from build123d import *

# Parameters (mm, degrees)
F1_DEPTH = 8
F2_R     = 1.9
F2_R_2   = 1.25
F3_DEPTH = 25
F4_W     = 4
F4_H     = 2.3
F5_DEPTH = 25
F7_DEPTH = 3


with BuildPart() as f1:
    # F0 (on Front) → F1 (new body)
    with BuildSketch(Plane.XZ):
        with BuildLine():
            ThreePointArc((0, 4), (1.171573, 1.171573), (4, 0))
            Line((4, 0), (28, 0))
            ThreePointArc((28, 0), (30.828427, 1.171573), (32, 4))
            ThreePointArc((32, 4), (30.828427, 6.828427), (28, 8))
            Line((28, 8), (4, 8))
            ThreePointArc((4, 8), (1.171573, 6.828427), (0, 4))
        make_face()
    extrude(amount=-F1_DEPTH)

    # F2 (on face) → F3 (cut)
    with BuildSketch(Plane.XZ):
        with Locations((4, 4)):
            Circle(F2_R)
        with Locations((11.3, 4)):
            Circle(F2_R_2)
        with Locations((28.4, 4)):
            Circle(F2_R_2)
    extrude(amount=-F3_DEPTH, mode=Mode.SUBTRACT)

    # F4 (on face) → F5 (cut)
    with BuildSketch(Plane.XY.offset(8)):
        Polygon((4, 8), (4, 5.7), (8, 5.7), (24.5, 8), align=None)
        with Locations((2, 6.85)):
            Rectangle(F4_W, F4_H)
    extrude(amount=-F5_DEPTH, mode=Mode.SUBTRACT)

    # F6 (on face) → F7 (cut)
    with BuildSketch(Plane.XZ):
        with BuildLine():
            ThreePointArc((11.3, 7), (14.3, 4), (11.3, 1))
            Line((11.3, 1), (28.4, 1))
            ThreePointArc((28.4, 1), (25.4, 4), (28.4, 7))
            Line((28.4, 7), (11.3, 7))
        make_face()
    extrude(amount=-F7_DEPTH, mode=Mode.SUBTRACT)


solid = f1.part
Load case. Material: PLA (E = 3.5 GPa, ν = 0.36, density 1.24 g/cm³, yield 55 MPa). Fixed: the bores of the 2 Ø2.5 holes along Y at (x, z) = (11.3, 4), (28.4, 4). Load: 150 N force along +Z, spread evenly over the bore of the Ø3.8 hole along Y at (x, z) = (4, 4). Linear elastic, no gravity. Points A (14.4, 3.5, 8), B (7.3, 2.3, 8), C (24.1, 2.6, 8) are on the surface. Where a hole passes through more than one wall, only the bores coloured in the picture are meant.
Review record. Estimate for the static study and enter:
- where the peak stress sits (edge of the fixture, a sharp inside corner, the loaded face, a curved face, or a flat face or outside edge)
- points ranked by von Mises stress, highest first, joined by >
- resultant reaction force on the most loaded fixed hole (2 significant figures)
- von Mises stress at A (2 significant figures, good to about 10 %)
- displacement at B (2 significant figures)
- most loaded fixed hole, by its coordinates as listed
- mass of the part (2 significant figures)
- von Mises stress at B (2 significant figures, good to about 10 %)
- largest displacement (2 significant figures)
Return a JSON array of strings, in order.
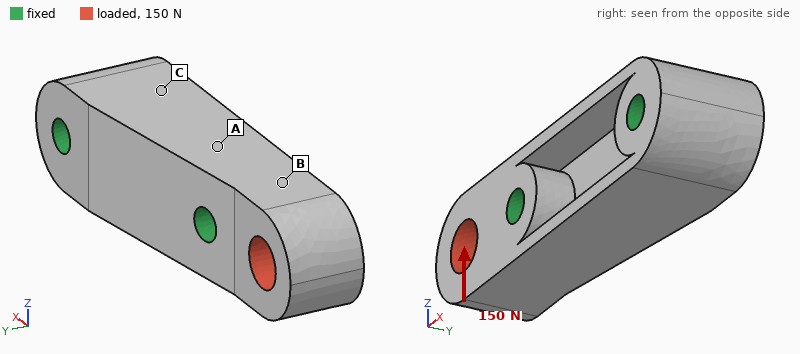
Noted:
["edge of the fixture", "B > A > C", "180 N", "6.3 MPa", "0.044 mm", "(11.3, 4)", "1.6 g", "12 MPa", "0.12 mm"]
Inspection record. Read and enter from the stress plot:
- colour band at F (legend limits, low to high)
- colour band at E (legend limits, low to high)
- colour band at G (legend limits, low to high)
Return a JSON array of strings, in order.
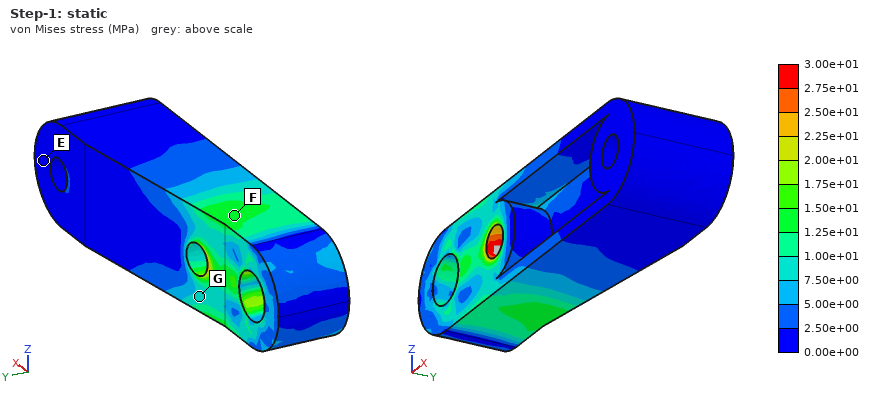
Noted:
["1.25e+01 to 1.50e+01 MPa", "0.00e+00 to 2.50e+00 MPa", "7.50e+00 to 1.00e+01 MPa"]
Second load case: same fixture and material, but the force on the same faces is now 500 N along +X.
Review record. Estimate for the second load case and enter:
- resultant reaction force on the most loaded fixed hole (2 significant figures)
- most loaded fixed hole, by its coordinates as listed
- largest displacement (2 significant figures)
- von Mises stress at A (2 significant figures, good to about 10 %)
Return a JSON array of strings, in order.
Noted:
["470 N", "(11.3, 4)", "54 µm", "3.1 MPa"]
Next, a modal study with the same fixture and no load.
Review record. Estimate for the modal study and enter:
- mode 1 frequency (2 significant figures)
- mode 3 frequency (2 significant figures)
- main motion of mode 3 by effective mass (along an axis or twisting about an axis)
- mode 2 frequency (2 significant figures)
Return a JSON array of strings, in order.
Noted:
["12 kHz", "18 kHz", "along Z", "13 kHz"]
